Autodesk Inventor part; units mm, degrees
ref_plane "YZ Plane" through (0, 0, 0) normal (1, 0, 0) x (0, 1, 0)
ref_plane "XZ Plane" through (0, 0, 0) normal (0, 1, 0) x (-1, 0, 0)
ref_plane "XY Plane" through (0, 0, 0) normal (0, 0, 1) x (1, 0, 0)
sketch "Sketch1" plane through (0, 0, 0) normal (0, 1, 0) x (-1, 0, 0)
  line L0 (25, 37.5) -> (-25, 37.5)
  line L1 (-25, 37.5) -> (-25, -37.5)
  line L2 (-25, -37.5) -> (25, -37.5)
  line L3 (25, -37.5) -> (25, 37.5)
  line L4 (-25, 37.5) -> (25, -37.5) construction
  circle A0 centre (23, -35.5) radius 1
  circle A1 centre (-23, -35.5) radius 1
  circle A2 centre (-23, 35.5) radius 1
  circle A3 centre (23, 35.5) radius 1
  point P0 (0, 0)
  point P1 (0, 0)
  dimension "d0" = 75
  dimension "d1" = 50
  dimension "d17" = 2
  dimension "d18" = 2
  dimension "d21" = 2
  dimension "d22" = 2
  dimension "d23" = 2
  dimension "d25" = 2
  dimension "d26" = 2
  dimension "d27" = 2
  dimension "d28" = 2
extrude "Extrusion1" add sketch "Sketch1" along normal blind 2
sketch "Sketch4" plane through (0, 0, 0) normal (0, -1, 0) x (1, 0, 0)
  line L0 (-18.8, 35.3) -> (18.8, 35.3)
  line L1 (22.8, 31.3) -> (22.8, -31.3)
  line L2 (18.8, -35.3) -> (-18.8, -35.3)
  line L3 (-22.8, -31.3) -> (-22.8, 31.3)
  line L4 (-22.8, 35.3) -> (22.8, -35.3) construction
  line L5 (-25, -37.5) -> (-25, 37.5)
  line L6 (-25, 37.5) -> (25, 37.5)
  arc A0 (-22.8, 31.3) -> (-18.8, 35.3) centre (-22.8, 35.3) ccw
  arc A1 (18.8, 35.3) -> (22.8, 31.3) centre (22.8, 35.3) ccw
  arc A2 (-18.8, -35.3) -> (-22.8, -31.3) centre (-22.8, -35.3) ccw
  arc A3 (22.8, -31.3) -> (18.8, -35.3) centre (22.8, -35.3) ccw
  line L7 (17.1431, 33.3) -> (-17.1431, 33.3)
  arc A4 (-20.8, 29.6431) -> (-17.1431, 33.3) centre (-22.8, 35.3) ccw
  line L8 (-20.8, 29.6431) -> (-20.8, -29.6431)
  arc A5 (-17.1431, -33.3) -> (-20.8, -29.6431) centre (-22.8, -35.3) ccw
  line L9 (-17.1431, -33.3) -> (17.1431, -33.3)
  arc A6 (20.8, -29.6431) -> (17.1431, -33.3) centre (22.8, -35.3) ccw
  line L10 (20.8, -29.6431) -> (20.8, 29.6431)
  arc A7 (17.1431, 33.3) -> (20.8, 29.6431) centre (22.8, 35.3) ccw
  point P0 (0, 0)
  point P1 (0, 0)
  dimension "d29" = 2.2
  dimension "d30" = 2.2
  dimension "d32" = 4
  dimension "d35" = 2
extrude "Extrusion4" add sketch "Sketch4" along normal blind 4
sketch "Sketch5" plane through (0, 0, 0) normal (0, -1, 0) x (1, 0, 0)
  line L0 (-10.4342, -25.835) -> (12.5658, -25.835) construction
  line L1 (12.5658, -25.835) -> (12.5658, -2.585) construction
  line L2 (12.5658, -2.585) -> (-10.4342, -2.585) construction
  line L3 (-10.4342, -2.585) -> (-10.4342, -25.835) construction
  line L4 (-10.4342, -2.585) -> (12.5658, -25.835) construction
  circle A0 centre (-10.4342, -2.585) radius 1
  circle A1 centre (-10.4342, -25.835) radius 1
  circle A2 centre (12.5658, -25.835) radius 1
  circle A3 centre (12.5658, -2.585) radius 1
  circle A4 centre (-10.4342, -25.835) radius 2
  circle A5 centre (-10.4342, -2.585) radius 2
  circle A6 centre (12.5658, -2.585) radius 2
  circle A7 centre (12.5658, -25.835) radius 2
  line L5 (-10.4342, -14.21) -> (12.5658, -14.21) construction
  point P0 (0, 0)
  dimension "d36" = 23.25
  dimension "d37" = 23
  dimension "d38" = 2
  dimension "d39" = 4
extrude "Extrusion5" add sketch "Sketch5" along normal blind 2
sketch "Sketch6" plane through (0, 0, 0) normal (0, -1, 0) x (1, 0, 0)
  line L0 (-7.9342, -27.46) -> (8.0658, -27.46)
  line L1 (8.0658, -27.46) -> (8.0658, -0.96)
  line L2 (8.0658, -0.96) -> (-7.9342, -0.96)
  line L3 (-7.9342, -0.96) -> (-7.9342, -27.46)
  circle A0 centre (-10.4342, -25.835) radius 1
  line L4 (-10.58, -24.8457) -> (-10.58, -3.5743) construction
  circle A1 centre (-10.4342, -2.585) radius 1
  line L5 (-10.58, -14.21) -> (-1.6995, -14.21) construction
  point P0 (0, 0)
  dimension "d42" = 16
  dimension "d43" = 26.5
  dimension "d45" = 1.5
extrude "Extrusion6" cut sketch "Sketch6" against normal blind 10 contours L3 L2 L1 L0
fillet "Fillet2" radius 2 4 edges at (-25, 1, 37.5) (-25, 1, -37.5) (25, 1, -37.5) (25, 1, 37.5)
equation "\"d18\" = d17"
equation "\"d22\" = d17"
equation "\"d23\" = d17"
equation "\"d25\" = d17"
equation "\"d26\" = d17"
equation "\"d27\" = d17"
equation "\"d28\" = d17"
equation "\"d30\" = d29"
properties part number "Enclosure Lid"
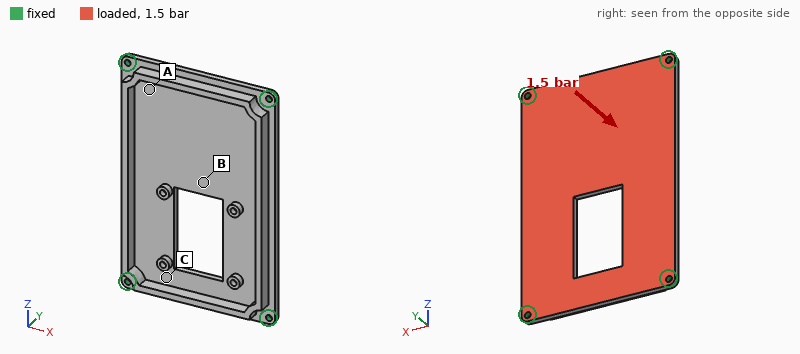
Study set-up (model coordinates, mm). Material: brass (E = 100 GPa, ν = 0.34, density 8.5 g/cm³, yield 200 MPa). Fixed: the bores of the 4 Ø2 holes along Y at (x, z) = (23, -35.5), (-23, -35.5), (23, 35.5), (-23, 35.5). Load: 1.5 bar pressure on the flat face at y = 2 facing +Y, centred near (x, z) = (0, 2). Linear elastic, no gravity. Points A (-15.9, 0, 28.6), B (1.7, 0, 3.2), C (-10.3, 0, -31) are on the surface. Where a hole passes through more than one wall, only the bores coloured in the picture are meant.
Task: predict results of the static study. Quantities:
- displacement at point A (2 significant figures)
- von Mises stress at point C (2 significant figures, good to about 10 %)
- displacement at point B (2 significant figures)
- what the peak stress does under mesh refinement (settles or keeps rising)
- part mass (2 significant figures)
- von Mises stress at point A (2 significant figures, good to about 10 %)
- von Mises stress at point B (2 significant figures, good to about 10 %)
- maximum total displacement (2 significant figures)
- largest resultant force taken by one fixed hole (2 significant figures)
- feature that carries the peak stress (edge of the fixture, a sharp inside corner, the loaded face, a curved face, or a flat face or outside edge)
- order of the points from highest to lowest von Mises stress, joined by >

0.027 mm
18 MPa
0.12 mm
keeps rising
72 g
9.8 MPa
28 MPa
0.13 mm
200 N
edge of the fixture
B > C > A
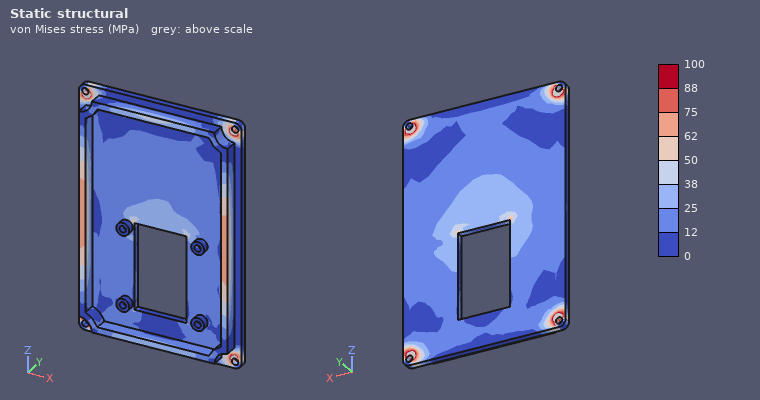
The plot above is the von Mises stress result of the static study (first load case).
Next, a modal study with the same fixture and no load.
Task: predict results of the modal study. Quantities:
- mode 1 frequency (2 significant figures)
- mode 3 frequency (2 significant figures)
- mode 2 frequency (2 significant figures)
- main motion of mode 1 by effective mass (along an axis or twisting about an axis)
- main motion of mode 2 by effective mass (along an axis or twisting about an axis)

1600 Hz
3800 Hz
2500 Hz
along Y
twisting about Z
